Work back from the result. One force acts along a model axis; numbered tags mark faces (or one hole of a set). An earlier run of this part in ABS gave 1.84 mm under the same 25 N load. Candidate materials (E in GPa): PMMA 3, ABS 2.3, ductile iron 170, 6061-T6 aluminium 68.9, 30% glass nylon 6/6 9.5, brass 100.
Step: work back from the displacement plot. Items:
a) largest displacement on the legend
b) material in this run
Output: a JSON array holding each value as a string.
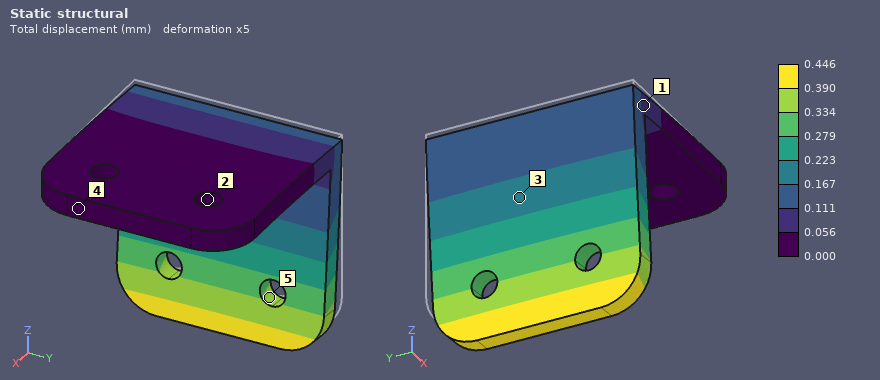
["0.446 mm", "30% glass nylon 6/6"]
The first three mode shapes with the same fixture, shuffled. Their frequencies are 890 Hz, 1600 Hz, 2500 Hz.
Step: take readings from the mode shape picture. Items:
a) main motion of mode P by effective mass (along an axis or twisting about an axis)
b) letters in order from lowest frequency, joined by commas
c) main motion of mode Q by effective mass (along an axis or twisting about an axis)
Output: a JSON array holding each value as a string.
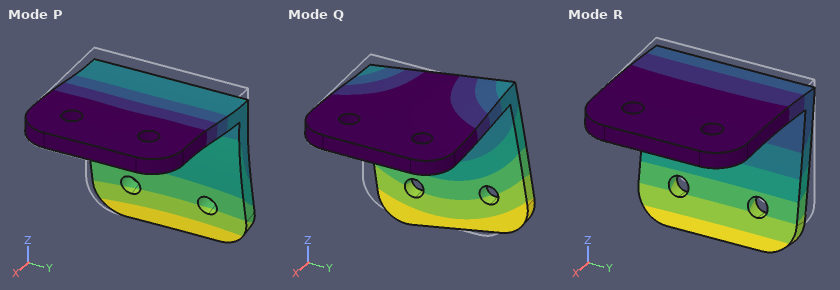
["along Z", "R, Q, P", "along Y"]
